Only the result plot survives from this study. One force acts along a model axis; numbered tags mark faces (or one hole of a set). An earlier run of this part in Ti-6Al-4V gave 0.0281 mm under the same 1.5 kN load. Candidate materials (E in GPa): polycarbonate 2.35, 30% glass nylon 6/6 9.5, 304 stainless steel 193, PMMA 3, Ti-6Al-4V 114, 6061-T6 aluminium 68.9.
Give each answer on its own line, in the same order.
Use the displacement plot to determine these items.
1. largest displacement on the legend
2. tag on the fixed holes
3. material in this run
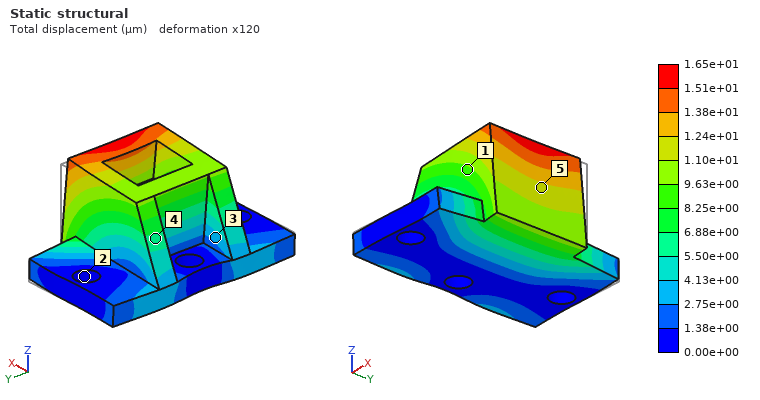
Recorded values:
1.65e+01 µm
2
304 stainless steel
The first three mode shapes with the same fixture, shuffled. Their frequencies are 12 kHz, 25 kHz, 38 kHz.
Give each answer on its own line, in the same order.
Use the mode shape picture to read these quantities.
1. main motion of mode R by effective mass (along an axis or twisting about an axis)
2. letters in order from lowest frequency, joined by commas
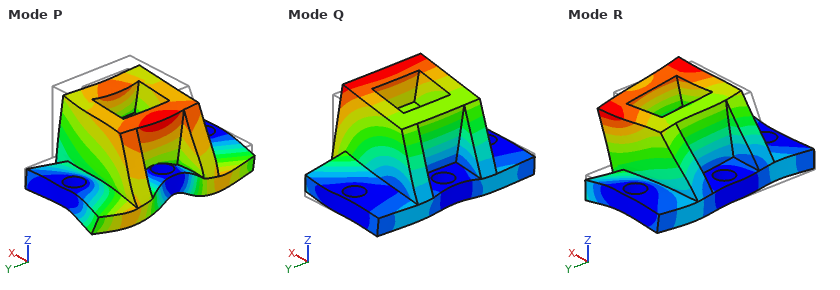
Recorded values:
along Y
Q, R, P
